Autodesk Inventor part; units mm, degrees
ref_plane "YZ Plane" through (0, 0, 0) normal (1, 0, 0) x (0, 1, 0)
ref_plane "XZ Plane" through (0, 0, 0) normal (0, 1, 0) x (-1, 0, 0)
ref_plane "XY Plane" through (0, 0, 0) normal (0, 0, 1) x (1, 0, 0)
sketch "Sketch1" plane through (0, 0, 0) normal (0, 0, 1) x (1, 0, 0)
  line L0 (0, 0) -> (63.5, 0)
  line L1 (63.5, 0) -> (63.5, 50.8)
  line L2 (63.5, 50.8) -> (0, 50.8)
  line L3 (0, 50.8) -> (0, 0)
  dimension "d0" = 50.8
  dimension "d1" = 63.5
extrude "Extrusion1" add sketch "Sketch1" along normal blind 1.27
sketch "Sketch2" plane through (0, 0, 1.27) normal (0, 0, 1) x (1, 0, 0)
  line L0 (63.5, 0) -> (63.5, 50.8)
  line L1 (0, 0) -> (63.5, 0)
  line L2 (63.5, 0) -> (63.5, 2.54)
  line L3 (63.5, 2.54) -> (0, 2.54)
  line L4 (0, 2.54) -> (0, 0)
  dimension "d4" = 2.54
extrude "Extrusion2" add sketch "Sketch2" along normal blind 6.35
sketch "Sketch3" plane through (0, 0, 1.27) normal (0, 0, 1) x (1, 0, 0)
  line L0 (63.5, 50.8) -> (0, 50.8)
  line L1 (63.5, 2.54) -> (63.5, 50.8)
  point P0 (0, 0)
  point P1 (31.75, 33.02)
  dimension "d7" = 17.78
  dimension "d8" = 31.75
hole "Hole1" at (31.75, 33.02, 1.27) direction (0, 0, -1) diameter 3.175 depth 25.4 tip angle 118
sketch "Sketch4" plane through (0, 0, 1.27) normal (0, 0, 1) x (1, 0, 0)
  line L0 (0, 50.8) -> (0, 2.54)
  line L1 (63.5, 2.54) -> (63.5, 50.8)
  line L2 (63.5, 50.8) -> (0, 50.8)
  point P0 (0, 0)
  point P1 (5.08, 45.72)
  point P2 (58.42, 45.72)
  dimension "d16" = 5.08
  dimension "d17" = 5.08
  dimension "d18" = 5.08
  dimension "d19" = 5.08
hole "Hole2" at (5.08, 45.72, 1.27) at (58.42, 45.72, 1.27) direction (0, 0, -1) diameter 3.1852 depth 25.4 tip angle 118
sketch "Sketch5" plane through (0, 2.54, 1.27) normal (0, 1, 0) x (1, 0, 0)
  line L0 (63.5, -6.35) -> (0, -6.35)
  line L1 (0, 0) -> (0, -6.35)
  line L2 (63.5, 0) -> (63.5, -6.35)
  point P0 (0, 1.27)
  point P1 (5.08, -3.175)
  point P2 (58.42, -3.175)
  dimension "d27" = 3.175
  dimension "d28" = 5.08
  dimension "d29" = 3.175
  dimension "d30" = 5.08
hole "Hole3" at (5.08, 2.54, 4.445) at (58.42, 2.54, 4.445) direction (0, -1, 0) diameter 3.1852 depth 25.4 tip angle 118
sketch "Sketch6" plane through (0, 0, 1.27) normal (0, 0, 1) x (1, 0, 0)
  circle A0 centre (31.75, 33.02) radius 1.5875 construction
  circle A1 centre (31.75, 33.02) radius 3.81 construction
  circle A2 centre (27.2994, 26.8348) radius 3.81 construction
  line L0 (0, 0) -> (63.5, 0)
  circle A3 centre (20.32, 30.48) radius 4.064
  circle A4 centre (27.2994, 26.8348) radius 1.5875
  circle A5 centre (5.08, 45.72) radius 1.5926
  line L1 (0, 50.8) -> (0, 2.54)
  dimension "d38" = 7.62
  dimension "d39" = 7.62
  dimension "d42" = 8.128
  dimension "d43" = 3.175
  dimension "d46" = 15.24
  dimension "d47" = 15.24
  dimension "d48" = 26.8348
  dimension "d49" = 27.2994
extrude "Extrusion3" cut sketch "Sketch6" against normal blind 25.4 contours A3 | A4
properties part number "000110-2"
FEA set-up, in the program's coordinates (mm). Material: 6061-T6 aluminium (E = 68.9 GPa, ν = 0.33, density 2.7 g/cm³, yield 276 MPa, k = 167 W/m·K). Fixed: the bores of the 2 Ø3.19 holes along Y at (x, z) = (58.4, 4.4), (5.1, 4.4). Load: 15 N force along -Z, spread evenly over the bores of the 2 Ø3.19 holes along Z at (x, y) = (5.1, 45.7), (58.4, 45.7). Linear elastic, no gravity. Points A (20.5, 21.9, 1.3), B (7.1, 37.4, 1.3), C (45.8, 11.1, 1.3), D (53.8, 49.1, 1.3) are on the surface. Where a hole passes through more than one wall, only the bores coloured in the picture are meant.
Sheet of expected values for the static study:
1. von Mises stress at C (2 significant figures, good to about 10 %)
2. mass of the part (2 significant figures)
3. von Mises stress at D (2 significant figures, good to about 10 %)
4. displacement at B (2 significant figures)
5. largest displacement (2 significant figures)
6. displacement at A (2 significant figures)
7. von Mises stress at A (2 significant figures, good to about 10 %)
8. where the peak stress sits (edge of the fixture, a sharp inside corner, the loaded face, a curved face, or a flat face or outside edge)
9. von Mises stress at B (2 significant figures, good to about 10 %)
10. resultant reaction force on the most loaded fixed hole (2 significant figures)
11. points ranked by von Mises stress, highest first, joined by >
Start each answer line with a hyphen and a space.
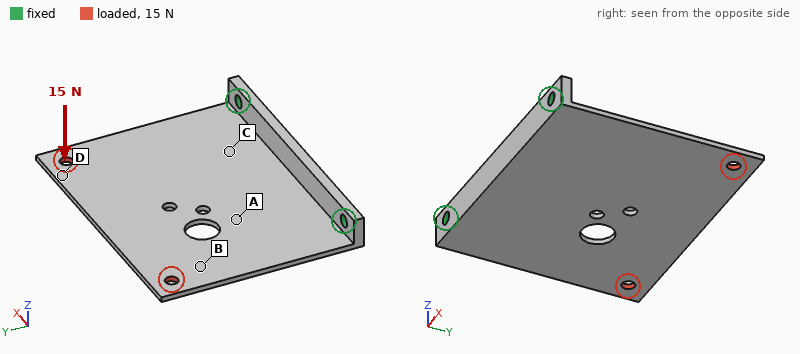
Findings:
- 27 MPa
- 13 g
- 4.5 MPa
- 0.44 mm
- 0.74 mm
- 0.17 mm
- 16 MPa
- a flat face or outside edge
- 10 MPa
- 7.6 N
- C > A > B > D
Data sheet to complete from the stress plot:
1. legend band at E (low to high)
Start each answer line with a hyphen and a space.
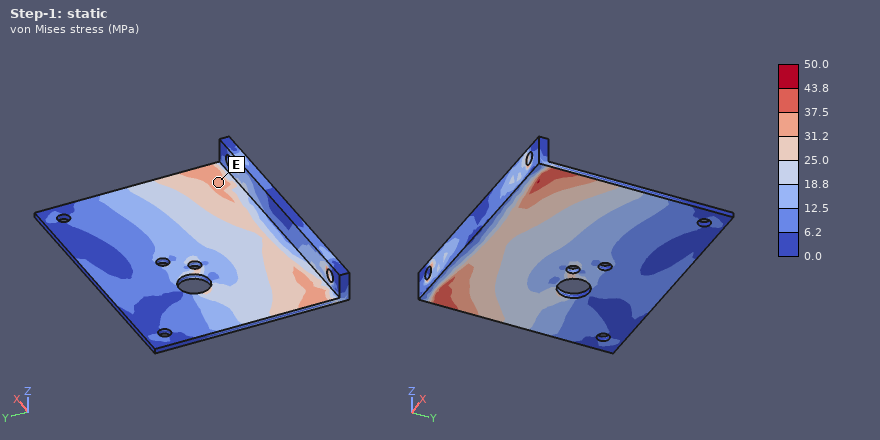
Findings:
- 31.2 to 37.5 MPa
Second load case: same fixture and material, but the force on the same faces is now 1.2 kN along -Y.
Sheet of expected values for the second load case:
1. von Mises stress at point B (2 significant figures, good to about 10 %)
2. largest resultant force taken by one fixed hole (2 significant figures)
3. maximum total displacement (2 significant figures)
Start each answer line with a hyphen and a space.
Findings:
- 34 MPa
- 610 N
- 0.16 mm
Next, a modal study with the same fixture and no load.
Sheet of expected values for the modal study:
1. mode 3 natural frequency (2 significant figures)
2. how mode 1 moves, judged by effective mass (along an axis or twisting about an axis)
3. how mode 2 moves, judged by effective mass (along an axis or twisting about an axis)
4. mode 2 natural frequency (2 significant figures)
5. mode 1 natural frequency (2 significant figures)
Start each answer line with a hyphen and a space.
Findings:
- 2200 Hz
- along Z
- twisting about Y
- 890 Hz
- 420 Hz
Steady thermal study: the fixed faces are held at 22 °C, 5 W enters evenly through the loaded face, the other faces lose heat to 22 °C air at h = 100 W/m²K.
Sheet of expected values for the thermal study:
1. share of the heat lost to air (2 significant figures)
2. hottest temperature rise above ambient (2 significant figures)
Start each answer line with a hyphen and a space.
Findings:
- 69 %
- 16 K
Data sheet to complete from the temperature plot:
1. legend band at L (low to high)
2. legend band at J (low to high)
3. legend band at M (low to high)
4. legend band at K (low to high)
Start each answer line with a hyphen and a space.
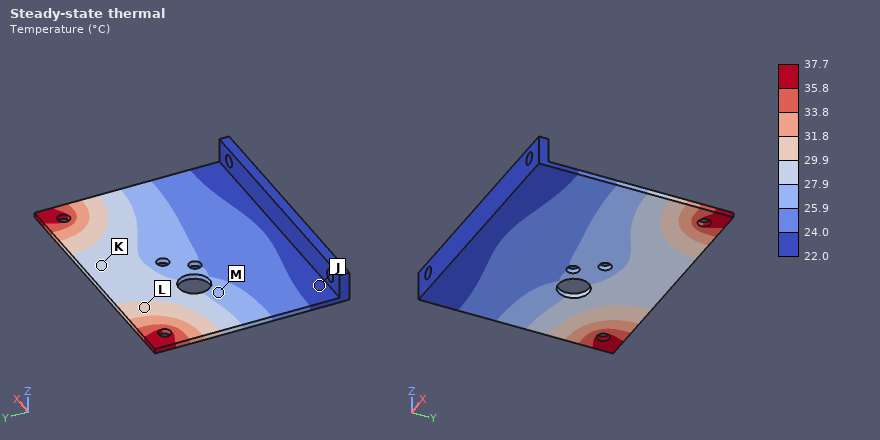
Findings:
- 29.9 to 31.8 °C
- 22.0 to 24.0 °C
- 25.9 to 27.9 °C
- 27.9 to 29.9 °C
